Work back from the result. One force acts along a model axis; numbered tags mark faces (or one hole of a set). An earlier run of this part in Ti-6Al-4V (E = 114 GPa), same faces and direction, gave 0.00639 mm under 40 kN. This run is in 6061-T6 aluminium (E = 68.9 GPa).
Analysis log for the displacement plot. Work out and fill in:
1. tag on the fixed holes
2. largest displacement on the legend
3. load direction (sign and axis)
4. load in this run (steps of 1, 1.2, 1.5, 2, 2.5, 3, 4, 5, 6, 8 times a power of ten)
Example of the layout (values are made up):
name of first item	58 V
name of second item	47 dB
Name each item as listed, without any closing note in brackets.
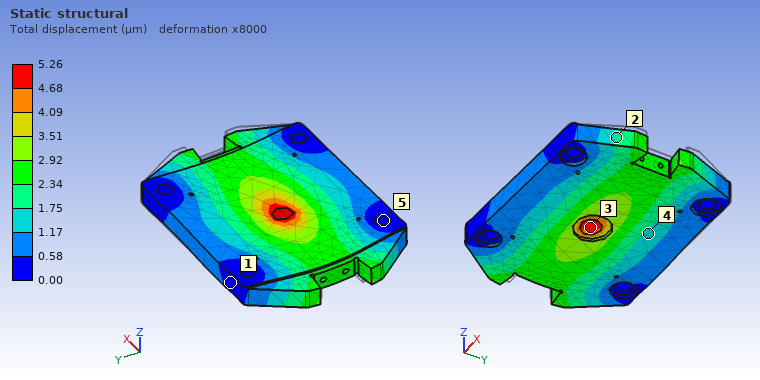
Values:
tag on the fixed holes	5
largest displacement on the legend	5.26 µm
load direction	-X
load in this run	20 kN
